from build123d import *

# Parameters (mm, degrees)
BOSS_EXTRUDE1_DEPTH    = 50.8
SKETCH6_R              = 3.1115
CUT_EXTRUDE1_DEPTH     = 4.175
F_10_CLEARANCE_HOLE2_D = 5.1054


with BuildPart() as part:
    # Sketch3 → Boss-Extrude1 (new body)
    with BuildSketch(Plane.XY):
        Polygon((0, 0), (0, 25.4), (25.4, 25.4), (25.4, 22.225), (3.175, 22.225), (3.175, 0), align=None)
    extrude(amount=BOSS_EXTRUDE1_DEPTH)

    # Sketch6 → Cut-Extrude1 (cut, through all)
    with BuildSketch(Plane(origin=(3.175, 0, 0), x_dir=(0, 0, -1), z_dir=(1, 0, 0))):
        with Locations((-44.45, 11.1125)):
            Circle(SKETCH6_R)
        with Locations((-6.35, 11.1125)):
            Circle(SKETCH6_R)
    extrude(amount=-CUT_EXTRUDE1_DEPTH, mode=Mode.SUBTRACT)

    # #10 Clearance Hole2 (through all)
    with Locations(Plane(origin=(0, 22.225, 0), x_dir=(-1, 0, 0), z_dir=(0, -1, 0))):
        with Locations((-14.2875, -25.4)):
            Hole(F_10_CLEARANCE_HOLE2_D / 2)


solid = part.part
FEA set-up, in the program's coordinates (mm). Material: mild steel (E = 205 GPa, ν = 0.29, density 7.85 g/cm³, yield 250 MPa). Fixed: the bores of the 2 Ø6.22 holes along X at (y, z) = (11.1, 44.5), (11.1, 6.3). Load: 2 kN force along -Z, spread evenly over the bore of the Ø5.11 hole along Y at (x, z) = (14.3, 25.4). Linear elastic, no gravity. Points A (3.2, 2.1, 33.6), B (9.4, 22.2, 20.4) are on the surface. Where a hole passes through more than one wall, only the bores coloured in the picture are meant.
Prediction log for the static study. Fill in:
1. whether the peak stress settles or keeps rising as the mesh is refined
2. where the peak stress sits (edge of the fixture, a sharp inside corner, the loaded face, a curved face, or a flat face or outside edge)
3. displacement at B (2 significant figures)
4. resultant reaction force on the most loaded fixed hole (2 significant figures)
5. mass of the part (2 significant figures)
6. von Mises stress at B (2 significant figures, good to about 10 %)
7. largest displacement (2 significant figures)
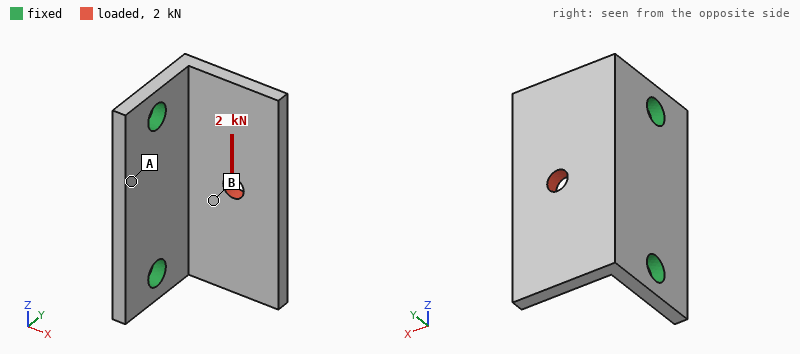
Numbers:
keeps rising
edge of the fixture
13 µm
1.3 kN
58 g
59 MPa
50 µm
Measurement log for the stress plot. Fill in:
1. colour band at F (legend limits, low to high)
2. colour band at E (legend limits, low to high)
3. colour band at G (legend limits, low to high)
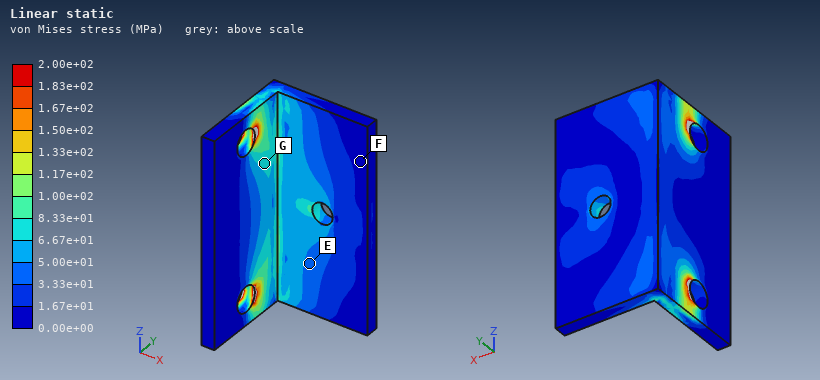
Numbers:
0.00e+00 to 1.67e+01 MPa
3.33e+01 to 5.00e+01 MPa
6.67e+01 to 8.33e+01 MPa
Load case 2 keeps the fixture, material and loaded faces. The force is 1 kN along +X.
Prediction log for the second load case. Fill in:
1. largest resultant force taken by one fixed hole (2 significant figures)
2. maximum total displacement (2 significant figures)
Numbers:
510 N
67 µm
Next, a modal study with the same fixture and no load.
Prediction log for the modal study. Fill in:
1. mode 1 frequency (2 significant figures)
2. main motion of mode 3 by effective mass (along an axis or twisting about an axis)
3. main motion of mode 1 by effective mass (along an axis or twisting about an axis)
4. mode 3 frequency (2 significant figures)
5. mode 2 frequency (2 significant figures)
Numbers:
2600 Hz
along X
along Y
8200 Hz
4900 Hz
